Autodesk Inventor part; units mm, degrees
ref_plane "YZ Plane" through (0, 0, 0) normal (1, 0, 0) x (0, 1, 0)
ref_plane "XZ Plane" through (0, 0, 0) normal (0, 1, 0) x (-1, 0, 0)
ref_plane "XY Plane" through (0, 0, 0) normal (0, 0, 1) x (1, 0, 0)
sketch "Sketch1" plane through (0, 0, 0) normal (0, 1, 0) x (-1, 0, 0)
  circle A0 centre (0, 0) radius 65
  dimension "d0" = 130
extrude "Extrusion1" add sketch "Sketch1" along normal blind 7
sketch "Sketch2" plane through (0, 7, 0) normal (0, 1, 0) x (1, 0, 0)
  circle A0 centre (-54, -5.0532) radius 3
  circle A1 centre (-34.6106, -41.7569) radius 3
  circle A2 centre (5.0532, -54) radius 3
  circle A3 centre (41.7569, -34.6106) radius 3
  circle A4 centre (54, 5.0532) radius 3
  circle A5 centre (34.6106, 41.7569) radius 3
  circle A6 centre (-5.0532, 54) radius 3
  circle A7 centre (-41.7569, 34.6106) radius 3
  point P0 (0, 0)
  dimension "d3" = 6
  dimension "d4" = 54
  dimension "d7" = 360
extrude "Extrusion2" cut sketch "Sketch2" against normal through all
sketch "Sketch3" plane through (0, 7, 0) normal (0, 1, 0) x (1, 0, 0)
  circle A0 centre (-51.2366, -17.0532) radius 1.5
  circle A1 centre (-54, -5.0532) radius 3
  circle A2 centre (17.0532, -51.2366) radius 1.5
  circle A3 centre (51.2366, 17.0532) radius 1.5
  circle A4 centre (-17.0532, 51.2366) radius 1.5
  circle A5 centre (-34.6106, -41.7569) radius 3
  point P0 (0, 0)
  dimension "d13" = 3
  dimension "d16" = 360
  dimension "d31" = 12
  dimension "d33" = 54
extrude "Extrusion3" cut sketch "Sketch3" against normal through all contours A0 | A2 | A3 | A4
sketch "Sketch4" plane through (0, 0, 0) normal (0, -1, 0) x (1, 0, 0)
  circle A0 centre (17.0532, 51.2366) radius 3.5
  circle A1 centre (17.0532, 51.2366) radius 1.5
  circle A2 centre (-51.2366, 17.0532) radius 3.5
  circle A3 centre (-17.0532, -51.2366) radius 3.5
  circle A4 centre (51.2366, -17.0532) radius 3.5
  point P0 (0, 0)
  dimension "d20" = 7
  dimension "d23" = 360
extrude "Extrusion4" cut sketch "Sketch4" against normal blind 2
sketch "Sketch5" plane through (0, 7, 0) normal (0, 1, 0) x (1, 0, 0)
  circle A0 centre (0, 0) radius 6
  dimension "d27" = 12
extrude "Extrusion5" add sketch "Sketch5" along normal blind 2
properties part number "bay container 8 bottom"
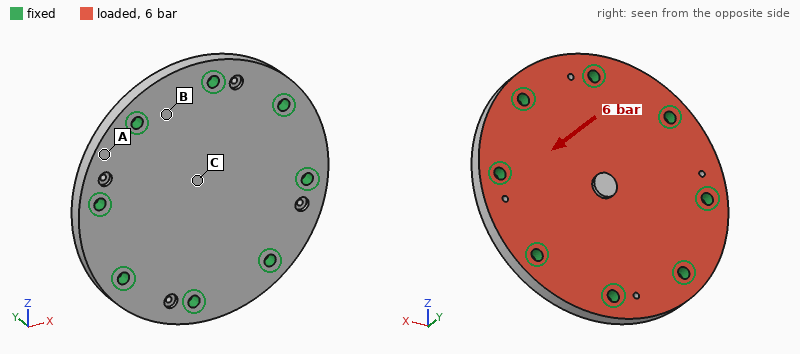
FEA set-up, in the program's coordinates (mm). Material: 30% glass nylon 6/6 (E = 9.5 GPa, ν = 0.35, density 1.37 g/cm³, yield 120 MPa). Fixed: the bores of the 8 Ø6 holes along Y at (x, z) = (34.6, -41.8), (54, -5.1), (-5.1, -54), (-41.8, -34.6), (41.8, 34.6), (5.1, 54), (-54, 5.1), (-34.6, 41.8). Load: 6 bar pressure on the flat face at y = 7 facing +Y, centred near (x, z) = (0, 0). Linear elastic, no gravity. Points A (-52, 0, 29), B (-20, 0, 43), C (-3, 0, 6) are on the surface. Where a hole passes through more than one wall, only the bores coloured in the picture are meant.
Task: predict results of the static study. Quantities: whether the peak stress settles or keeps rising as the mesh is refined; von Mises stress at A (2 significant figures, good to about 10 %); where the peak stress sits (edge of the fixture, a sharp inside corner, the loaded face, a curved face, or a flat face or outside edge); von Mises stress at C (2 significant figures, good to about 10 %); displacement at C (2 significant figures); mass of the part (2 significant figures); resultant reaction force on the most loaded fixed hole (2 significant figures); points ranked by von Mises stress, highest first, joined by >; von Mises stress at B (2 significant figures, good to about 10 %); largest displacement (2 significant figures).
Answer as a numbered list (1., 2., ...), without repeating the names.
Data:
1. keeps rising
2. 4.8 MPa
3. edge of the fixture
4. 17 MPa
5. 0.30 mm
6. 120 g
7. 970 N
8. C > B > A
9. 12 MPa
10. 0.31 mm
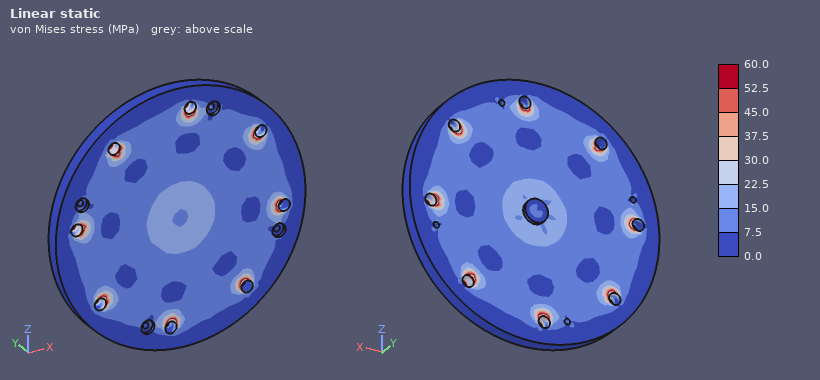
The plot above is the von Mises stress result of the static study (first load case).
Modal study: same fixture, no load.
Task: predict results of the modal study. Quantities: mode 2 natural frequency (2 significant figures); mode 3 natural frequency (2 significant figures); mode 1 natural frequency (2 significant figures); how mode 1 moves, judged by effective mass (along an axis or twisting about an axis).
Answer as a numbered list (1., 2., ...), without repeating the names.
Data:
1. 5400 Hz
2. 5400 Hz
3. 2700 Hz
4. along Y
